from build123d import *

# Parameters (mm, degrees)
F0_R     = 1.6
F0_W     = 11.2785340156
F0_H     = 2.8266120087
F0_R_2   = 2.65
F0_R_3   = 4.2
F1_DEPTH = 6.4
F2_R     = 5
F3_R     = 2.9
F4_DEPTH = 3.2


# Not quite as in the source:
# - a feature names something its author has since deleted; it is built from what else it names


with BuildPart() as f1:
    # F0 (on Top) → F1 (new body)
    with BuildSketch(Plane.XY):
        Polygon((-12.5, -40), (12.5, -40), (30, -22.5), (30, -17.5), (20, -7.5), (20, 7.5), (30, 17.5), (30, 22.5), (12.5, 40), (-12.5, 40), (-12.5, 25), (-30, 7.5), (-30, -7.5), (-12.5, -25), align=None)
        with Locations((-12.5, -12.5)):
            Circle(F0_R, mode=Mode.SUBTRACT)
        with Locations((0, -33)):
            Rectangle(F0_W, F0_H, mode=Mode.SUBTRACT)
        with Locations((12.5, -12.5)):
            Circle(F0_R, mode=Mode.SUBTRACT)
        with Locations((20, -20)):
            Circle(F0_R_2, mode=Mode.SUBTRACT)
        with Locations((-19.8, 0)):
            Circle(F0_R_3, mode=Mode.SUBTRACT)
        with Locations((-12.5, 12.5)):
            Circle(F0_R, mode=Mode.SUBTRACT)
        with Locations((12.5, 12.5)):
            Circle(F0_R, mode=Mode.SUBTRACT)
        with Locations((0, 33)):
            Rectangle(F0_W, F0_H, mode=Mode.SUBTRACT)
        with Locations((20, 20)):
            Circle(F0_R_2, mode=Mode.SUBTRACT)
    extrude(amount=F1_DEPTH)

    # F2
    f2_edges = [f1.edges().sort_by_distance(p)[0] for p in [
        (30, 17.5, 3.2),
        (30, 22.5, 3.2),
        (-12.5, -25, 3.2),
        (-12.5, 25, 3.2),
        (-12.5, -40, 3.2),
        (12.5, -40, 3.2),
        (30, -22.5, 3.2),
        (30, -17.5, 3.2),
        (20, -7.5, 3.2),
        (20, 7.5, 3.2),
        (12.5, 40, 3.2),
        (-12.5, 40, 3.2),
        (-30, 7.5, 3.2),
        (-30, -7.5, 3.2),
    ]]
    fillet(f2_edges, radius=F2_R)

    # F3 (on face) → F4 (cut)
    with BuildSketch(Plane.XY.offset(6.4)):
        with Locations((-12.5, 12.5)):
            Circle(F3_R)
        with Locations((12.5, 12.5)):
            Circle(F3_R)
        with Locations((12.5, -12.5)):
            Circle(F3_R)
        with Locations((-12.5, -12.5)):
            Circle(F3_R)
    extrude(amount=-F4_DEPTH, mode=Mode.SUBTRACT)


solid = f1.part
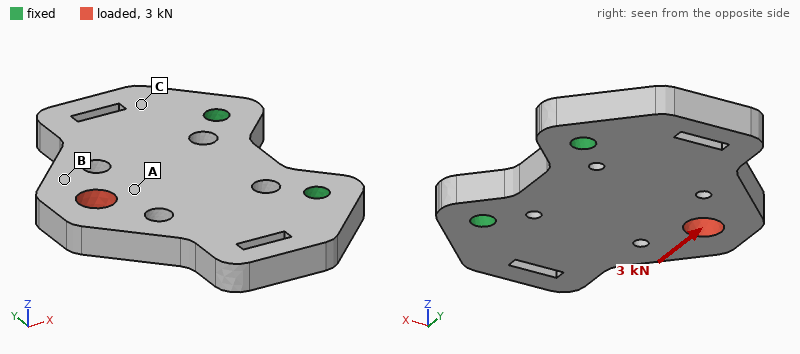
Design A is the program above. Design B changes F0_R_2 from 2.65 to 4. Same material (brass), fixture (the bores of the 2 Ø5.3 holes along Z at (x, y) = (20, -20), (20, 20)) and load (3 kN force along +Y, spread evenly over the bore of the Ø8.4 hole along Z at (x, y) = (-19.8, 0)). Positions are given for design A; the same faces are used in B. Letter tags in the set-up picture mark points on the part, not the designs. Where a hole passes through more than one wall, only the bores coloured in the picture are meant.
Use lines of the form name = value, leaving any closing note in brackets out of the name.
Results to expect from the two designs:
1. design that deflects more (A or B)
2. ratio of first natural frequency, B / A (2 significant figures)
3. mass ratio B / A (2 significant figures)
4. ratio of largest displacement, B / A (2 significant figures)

design that deflects more = A
ratio of first natural frequency, B / A = 1.1
mass ratio B / A = 0.98
ratio of largest displacement, B / A = 0.87
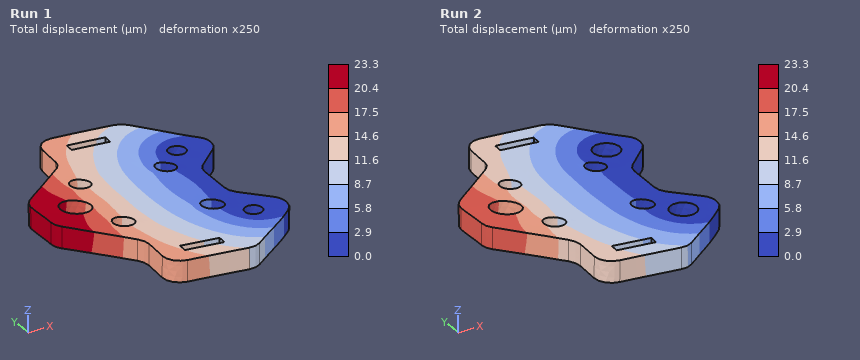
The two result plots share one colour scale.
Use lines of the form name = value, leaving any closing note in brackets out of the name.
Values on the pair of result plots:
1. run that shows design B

run that shows design B = Run 2
